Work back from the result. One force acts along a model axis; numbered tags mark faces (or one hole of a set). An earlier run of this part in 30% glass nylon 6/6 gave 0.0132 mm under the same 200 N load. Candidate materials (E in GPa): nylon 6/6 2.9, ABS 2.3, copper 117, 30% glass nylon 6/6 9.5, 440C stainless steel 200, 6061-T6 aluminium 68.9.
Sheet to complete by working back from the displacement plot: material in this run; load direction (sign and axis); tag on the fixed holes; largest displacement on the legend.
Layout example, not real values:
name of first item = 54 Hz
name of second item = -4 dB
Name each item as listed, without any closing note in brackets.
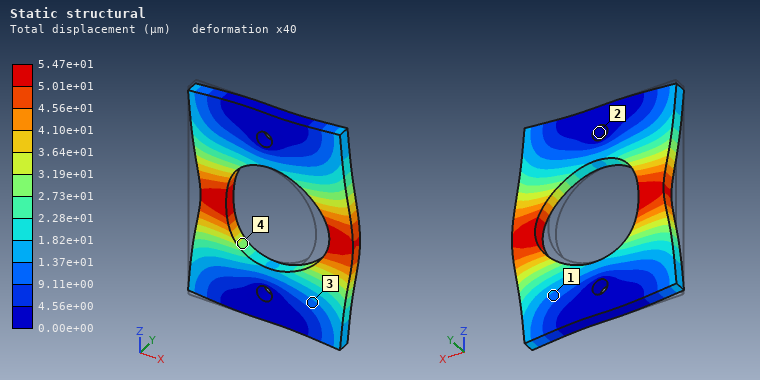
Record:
material in this run = ABS
load direction = +X
tag on the fixed holes = 2
largest displacement on the legend = 5.47e+01 µm
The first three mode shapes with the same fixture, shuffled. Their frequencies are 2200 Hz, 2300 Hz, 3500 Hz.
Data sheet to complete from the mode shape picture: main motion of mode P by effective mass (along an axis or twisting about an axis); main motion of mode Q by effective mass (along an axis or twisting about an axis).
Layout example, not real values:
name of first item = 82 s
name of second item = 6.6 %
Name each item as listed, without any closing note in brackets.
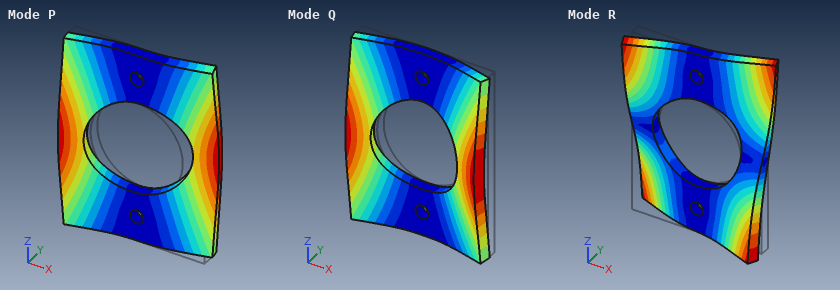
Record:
main motion of mode P by effective mass = twisting about Z
main motion of mode Q by effective mass = along Y
